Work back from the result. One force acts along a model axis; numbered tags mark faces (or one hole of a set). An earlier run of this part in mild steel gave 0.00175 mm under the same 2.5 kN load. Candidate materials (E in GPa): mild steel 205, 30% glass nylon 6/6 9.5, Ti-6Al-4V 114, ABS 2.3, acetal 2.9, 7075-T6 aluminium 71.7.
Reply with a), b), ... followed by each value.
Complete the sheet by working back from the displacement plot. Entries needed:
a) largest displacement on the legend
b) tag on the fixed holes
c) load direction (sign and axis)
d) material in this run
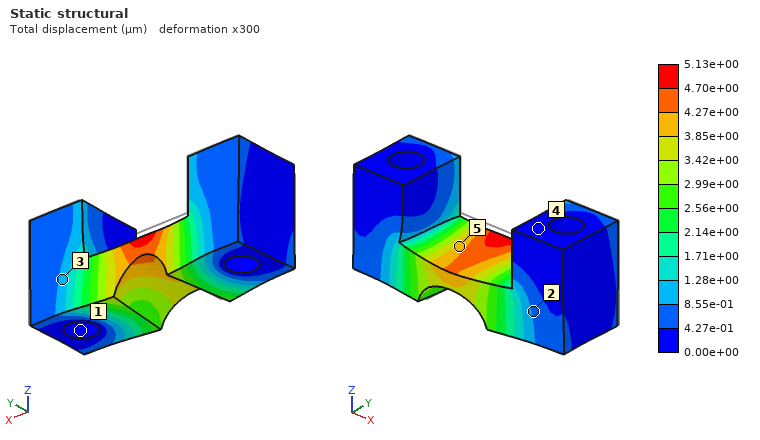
a) 5.13e+00 µm
b) 1
c) -Y
d) 7075-T6 aluminium
